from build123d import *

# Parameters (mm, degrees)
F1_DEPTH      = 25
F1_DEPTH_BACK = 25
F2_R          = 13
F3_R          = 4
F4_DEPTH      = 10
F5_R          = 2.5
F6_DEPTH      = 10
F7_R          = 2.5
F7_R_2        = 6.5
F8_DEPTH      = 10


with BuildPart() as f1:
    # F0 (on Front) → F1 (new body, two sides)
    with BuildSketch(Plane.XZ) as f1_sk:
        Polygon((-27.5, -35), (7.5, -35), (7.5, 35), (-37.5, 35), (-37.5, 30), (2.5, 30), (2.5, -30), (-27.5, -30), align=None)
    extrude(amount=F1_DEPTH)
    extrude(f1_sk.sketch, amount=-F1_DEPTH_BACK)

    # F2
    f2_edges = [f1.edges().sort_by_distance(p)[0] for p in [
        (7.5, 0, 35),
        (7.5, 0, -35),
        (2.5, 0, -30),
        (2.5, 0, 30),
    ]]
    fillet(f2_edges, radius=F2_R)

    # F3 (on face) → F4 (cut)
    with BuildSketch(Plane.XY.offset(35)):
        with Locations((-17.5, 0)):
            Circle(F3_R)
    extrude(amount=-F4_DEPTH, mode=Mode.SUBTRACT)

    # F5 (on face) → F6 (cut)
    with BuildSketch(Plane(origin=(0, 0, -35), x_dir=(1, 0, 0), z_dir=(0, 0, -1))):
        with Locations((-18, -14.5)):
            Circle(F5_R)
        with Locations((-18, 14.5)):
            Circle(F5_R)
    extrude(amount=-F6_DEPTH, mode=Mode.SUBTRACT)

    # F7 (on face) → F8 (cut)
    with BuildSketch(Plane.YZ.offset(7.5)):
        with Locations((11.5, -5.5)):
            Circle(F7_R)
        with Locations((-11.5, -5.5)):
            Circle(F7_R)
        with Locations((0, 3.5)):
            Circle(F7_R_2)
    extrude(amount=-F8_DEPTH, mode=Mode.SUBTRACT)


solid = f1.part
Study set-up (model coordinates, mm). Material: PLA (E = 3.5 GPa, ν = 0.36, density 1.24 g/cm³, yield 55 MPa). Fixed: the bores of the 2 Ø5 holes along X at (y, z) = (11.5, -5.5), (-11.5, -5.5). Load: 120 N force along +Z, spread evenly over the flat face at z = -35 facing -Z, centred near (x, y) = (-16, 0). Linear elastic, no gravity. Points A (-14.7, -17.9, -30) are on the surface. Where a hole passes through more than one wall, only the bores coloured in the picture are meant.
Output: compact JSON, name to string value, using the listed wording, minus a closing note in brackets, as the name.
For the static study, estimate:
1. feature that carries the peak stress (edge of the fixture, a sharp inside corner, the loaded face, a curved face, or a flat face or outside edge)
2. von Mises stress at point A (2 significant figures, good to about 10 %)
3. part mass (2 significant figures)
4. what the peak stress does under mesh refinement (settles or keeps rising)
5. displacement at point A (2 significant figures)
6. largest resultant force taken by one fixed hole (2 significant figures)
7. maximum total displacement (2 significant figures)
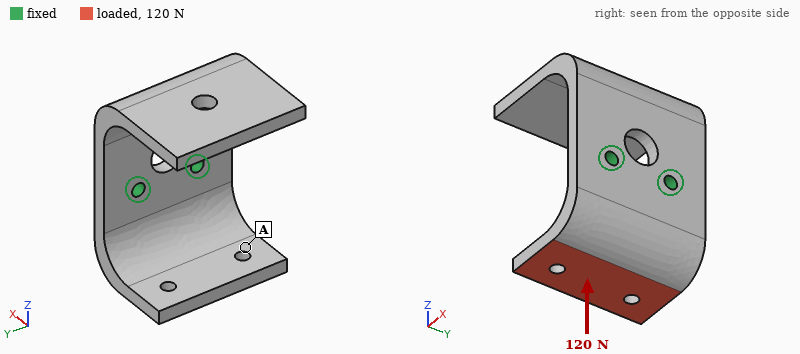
{"feature that carries the peak stress": "edge of the fixture", "von Mises stress at point A": "2.5 MPa", "part mass": "42 g", "what the peak stress does under mesh refinement": "keeps rising", "displacement at point A": "0.65 mm", "largest resultant force taken by one fixed hole": "63 N", "maximum total displacement": "1.1 mm"}
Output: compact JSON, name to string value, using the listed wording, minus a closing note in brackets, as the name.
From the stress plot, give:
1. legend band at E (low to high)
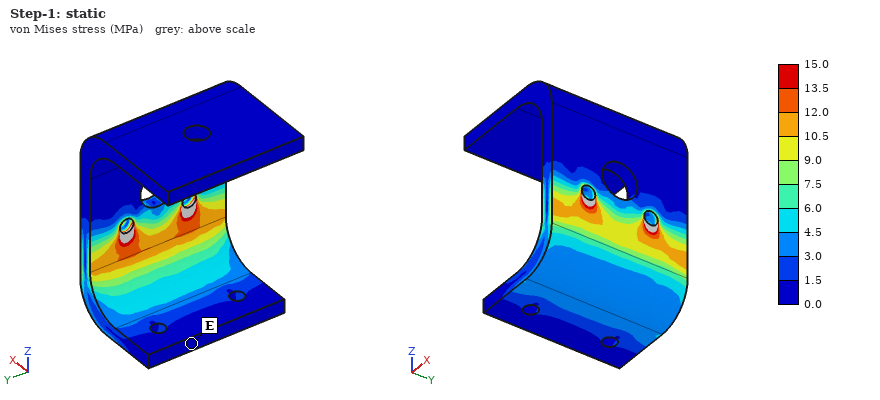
{"legend band at E": "0.0 to 1.5 MPa"}
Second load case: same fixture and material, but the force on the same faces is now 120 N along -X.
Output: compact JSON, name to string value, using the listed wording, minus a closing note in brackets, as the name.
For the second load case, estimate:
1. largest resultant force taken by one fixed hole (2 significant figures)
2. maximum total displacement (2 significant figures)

{"largest resultant force taken by one fixed hole": "60 N", "maximum total displacement": "0.96 mm"}
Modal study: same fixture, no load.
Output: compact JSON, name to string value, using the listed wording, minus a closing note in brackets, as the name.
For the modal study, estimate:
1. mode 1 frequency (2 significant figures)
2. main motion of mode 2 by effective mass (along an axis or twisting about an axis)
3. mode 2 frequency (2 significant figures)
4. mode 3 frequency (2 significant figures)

{"mode 1 frequency": "280 Hz", "main motion of mode 2 by effective mass": "along Y", "mode 2 frequency": "560 Hz", "mode 3 frequency": "600 Hz"}
